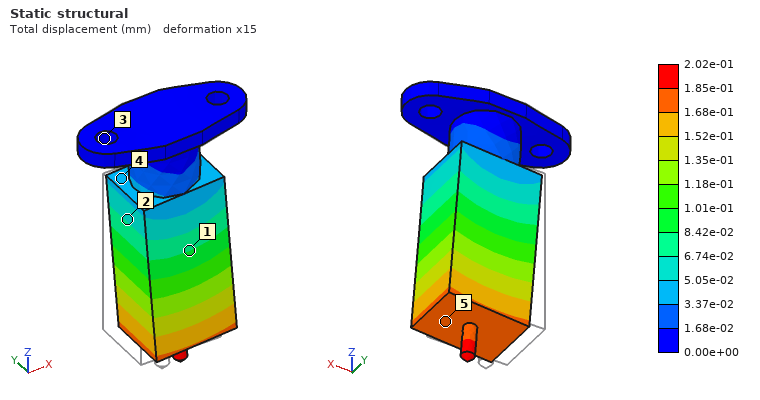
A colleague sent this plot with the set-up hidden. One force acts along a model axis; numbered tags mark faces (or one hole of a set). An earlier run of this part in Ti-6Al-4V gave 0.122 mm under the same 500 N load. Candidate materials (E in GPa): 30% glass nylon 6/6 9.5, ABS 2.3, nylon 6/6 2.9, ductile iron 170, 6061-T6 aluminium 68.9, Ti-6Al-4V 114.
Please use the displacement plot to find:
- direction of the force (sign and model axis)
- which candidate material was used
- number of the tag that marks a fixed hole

+X
6061-T6 aluminium
3
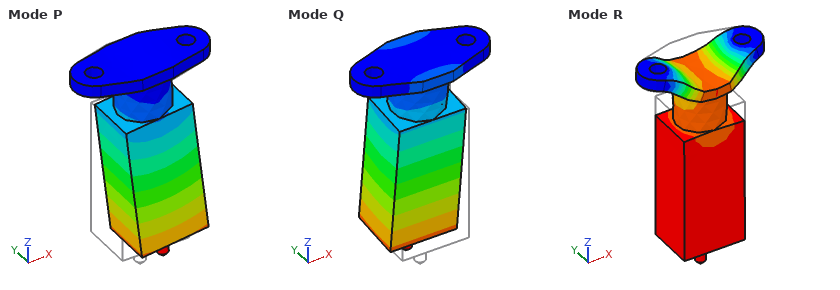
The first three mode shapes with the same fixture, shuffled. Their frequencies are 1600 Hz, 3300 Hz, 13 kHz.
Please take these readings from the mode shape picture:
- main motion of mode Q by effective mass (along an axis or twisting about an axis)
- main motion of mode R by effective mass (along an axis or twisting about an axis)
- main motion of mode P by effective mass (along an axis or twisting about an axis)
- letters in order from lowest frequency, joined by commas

along Y
along Z
along X
Q, P, R
